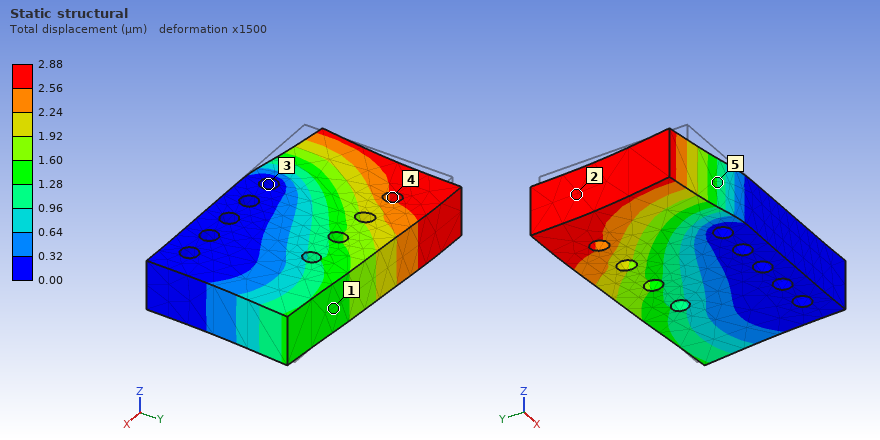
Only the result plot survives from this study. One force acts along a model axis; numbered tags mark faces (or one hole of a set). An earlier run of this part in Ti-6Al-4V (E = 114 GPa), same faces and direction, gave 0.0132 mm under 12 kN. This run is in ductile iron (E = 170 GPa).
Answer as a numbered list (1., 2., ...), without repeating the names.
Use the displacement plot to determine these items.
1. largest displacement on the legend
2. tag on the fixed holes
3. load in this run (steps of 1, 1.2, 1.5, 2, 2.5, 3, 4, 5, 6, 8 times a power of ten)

1. 2.88 µm
2. 3
3. 4 kN
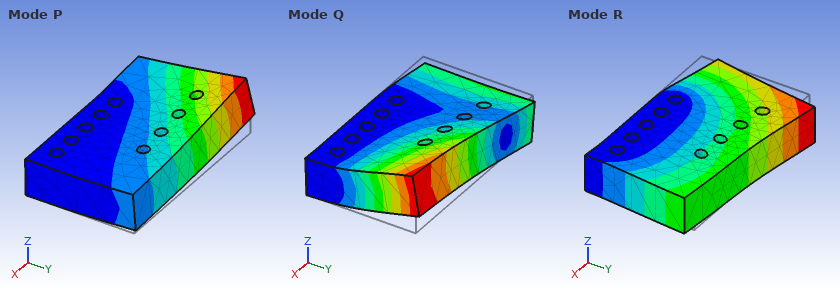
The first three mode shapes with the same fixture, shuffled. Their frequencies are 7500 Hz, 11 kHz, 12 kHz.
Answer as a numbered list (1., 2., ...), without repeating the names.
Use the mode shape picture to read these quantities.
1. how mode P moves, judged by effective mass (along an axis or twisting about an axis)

1. along Z
